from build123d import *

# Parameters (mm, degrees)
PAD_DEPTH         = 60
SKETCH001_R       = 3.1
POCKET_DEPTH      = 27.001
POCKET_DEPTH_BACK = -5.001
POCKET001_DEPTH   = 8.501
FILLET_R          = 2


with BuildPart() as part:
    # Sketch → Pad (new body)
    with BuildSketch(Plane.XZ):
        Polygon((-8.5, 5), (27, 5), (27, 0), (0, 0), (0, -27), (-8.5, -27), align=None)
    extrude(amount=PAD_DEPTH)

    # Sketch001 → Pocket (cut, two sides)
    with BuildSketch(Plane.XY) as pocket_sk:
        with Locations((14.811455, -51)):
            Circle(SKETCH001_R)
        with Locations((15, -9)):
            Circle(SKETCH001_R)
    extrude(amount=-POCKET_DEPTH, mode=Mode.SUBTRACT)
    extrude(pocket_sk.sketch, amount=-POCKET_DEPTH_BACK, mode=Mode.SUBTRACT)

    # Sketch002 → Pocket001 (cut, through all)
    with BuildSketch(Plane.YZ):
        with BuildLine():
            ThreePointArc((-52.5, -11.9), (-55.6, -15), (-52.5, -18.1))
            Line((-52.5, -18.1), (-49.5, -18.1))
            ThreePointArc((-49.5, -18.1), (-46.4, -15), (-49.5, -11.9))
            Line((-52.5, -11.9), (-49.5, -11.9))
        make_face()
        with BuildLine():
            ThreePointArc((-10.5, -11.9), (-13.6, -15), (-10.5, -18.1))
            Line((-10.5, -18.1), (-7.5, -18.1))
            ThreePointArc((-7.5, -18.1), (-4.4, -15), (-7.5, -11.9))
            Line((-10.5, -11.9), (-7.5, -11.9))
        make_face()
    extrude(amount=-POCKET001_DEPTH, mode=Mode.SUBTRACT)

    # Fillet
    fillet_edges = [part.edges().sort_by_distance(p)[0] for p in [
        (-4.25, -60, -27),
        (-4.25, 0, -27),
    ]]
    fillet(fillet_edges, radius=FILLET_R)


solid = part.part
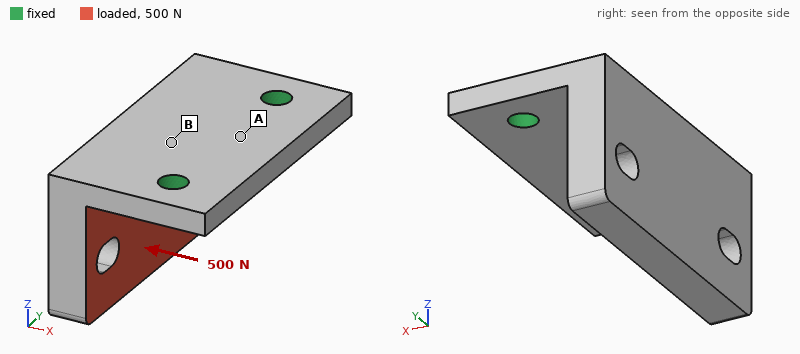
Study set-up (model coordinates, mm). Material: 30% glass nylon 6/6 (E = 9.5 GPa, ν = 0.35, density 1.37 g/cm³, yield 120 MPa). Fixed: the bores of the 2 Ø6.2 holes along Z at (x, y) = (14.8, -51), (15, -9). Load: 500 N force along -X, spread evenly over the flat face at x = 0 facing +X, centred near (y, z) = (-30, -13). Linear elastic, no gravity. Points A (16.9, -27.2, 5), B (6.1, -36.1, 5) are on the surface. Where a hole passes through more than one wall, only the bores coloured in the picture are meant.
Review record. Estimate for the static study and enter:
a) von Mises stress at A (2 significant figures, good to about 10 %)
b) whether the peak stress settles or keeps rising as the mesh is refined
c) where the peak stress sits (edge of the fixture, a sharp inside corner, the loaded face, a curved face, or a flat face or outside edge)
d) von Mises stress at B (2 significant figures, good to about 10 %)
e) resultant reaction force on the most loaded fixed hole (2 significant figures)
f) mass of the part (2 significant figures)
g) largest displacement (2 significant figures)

8.8 MPa
keeps rising
edge of the fixture
23 MPa
260 N
32 g
0.77 mm
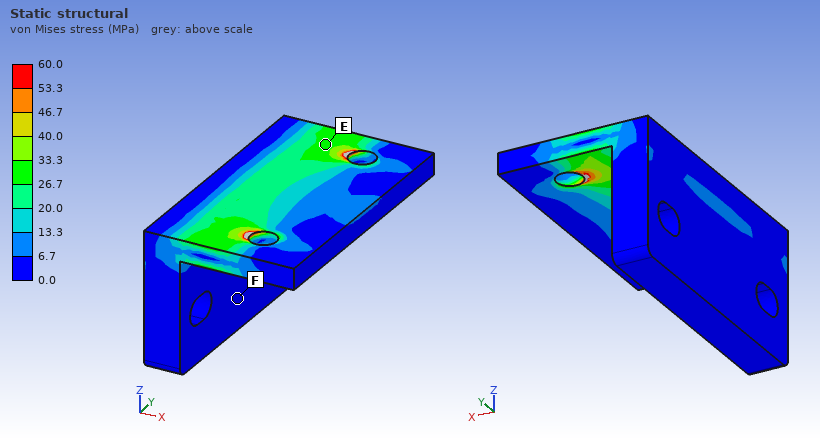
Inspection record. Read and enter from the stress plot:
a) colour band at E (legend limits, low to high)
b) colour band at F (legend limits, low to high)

26.7 to 33.3 MPa
0.0 to 6.7 MPa
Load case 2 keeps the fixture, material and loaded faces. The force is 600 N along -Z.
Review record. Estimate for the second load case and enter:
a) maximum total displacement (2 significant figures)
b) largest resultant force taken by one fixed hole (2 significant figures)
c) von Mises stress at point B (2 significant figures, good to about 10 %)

0.36 mm
300 N
8.7 MPa
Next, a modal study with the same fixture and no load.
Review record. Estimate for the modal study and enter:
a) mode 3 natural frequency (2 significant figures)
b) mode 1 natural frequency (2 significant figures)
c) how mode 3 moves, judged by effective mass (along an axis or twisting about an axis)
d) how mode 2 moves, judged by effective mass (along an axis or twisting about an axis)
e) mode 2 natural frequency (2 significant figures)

3600 Hz
1000 Hz
along Z
along Y
2400 Hz
